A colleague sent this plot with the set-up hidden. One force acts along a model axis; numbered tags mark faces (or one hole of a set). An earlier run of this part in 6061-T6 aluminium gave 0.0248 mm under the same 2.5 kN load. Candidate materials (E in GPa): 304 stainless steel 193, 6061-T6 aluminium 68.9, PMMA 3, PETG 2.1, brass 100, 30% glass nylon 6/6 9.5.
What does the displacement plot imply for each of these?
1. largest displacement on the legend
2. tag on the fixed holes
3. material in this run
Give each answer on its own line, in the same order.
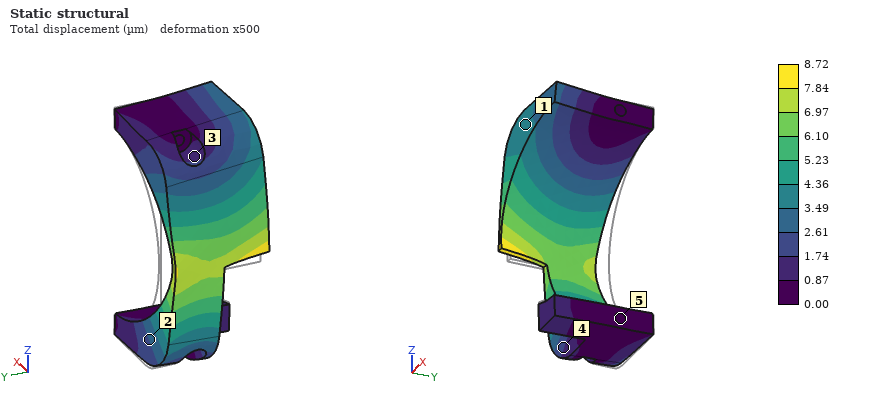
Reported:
8.72 µm
5
304 stainless steel
